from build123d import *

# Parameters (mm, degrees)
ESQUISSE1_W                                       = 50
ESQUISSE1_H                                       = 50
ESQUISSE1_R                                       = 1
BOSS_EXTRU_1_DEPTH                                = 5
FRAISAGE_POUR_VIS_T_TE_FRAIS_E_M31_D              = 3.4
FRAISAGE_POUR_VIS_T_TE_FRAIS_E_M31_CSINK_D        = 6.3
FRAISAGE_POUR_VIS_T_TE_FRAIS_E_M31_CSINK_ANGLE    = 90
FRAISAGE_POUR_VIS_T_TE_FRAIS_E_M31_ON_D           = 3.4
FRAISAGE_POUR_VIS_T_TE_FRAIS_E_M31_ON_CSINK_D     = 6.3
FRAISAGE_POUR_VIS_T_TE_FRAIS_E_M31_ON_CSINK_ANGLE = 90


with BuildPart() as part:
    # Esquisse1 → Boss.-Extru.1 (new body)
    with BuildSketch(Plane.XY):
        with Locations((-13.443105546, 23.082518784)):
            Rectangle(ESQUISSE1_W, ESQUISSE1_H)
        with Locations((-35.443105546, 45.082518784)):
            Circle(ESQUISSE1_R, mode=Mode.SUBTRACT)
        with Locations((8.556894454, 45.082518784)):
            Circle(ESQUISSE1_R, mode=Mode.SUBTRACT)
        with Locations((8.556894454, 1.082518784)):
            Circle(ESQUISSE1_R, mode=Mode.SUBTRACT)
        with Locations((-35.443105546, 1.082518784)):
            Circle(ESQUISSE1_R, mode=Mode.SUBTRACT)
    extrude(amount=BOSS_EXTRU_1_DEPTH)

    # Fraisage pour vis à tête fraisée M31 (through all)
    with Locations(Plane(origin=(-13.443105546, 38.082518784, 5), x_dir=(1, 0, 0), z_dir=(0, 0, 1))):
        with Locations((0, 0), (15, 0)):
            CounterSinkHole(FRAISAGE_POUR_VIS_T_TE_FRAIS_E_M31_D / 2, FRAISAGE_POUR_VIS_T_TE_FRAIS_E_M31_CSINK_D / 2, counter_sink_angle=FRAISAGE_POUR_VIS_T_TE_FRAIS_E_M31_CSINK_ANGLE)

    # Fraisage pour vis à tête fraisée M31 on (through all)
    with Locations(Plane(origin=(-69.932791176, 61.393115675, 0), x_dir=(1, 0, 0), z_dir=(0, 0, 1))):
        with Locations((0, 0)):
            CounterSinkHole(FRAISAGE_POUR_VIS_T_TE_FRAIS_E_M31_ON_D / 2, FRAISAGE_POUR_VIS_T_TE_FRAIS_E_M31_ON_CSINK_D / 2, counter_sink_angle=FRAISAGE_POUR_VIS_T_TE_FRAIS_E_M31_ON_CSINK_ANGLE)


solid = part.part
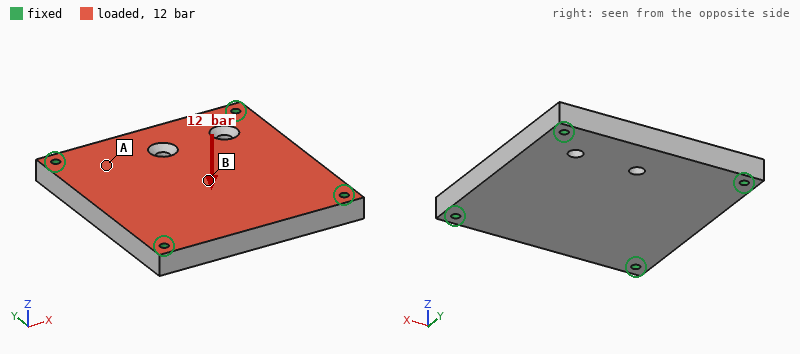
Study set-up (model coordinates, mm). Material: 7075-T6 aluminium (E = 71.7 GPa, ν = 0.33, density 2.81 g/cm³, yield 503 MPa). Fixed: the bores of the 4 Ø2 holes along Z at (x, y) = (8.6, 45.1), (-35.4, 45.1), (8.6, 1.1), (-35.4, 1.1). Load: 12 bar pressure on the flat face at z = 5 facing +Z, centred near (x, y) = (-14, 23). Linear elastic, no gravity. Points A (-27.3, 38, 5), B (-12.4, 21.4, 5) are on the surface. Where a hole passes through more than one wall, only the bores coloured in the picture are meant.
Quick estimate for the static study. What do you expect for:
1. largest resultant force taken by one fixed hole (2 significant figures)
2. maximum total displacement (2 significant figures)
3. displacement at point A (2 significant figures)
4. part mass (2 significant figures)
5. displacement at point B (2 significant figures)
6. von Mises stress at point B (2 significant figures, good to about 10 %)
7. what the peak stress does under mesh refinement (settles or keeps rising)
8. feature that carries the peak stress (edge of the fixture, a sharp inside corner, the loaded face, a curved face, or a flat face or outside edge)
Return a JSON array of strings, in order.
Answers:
["740 N", "55 µm", "28 µm", "35 g", "55 µm", "34 MPa", "keeps rising", "edge of the fixture"]
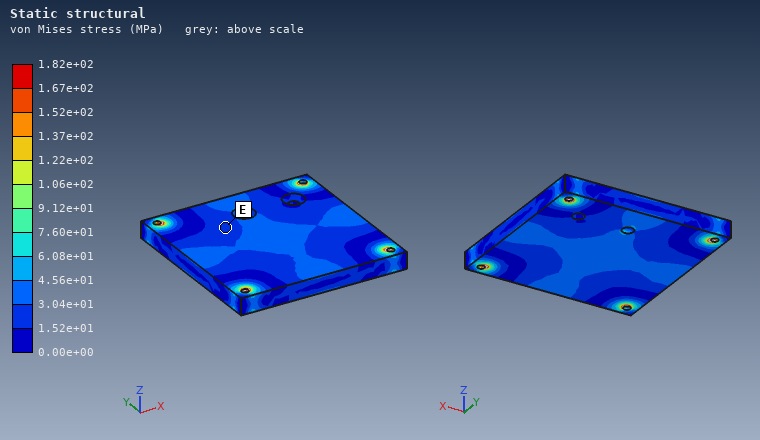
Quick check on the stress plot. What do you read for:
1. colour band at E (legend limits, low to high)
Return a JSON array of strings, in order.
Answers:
["1.52e+01 to 3.04e+01 MPa"]
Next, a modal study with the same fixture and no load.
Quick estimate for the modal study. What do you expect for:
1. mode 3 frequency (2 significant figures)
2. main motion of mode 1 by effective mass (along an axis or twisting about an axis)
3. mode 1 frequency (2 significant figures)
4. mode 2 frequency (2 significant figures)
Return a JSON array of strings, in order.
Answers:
["13 kHz", "along Z", "7300 Hz", "13 kHz"]
